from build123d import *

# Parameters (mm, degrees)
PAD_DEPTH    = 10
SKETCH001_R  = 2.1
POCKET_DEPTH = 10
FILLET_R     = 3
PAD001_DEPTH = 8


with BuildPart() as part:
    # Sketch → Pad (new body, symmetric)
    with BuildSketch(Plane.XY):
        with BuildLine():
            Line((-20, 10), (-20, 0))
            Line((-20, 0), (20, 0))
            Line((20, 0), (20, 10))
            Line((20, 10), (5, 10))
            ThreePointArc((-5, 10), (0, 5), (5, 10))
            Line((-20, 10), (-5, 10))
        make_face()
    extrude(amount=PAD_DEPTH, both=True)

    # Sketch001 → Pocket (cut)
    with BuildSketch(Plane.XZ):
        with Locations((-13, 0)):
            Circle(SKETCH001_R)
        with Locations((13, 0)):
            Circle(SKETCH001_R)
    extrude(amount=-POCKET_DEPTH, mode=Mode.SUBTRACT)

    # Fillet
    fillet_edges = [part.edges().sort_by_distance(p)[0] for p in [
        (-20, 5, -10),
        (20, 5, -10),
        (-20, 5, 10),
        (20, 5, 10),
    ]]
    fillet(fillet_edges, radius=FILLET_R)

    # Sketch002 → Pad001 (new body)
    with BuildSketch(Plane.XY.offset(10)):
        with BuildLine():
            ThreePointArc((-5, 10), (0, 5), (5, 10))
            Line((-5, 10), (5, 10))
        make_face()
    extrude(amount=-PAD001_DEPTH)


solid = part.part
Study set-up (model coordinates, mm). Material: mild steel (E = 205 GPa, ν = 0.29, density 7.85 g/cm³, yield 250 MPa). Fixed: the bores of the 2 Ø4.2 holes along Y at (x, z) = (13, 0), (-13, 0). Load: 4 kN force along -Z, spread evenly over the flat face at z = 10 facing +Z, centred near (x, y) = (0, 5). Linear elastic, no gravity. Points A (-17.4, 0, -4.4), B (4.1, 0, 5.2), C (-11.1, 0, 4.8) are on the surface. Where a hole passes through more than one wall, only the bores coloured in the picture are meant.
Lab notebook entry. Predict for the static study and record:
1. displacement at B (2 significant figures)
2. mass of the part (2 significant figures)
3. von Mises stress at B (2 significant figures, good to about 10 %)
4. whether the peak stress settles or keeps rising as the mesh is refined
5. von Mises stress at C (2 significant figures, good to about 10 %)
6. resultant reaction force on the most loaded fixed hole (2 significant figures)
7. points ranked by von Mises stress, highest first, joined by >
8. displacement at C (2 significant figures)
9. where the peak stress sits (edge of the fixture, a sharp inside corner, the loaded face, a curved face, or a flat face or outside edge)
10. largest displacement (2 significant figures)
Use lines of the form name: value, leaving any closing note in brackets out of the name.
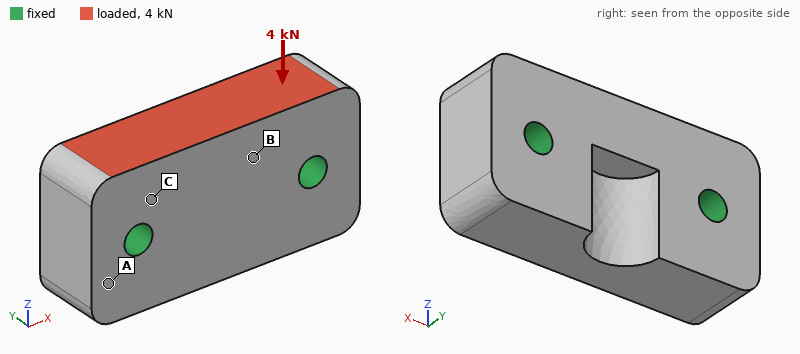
displacement at B: 1.1 µm
mass of the part: 56 g
von Mises stress at B: 9.8 MPa
whether the peak stress settles or keeps rising as the mesh is refined: keeps rising
von Mises stress at C: 17 MPa
resultant reaction force on the most loaded fixed hole: 2.0 kN
points ranked by von Mises stress, highest first, joined by >: C > B > A
displacement at C: 0.42 µm
where the peak stress sits: edge of the fixture
largest displacement: 1.6 µm
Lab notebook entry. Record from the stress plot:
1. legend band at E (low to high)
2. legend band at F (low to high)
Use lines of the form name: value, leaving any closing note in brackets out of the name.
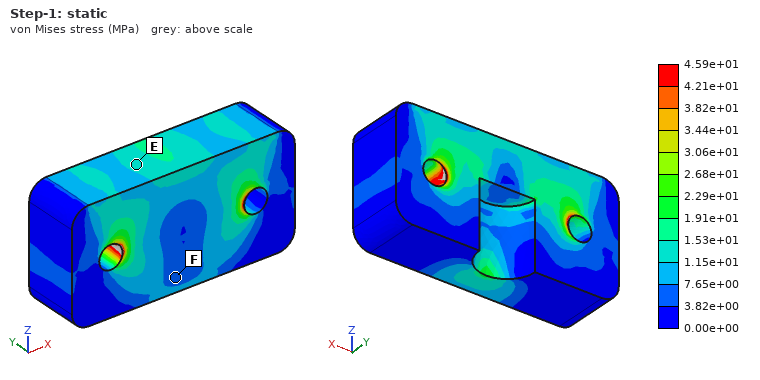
legend band at E: 1.15e+01 to 1.53e+01 MPa
legend band at F: 3.82e+00 to 7.65e+00 MPa
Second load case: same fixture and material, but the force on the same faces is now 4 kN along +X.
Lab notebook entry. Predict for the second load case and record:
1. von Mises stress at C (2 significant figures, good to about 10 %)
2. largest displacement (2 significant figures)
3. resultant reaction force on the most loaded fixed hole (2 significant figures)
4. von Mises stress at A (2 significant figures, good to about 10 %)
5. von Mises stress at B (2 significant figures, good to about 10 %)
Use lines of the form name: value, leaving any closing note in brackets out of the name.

von Mises stress at C: 23 MPa
largest displacement: 2.1 µm
resultant reaction force on the most loaded fixed hole: 2.4 kN
von Mises stress at A: 8.0 MPa
von Mises stress at B: 22 MPa
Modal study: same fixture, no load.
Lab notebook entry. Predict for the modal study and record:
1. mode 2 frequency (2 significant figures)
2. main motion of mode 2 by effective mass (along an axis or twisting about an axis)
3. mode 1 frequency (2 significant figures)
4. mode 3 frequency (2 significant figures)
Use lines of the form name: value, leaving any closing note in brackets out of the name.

mode 2 frequency: 40 kHz
main motion of mode 2 by effective mass: along Y
mode 1 frequency: 39 kHz
mode 3 frequency: 47 kHz
